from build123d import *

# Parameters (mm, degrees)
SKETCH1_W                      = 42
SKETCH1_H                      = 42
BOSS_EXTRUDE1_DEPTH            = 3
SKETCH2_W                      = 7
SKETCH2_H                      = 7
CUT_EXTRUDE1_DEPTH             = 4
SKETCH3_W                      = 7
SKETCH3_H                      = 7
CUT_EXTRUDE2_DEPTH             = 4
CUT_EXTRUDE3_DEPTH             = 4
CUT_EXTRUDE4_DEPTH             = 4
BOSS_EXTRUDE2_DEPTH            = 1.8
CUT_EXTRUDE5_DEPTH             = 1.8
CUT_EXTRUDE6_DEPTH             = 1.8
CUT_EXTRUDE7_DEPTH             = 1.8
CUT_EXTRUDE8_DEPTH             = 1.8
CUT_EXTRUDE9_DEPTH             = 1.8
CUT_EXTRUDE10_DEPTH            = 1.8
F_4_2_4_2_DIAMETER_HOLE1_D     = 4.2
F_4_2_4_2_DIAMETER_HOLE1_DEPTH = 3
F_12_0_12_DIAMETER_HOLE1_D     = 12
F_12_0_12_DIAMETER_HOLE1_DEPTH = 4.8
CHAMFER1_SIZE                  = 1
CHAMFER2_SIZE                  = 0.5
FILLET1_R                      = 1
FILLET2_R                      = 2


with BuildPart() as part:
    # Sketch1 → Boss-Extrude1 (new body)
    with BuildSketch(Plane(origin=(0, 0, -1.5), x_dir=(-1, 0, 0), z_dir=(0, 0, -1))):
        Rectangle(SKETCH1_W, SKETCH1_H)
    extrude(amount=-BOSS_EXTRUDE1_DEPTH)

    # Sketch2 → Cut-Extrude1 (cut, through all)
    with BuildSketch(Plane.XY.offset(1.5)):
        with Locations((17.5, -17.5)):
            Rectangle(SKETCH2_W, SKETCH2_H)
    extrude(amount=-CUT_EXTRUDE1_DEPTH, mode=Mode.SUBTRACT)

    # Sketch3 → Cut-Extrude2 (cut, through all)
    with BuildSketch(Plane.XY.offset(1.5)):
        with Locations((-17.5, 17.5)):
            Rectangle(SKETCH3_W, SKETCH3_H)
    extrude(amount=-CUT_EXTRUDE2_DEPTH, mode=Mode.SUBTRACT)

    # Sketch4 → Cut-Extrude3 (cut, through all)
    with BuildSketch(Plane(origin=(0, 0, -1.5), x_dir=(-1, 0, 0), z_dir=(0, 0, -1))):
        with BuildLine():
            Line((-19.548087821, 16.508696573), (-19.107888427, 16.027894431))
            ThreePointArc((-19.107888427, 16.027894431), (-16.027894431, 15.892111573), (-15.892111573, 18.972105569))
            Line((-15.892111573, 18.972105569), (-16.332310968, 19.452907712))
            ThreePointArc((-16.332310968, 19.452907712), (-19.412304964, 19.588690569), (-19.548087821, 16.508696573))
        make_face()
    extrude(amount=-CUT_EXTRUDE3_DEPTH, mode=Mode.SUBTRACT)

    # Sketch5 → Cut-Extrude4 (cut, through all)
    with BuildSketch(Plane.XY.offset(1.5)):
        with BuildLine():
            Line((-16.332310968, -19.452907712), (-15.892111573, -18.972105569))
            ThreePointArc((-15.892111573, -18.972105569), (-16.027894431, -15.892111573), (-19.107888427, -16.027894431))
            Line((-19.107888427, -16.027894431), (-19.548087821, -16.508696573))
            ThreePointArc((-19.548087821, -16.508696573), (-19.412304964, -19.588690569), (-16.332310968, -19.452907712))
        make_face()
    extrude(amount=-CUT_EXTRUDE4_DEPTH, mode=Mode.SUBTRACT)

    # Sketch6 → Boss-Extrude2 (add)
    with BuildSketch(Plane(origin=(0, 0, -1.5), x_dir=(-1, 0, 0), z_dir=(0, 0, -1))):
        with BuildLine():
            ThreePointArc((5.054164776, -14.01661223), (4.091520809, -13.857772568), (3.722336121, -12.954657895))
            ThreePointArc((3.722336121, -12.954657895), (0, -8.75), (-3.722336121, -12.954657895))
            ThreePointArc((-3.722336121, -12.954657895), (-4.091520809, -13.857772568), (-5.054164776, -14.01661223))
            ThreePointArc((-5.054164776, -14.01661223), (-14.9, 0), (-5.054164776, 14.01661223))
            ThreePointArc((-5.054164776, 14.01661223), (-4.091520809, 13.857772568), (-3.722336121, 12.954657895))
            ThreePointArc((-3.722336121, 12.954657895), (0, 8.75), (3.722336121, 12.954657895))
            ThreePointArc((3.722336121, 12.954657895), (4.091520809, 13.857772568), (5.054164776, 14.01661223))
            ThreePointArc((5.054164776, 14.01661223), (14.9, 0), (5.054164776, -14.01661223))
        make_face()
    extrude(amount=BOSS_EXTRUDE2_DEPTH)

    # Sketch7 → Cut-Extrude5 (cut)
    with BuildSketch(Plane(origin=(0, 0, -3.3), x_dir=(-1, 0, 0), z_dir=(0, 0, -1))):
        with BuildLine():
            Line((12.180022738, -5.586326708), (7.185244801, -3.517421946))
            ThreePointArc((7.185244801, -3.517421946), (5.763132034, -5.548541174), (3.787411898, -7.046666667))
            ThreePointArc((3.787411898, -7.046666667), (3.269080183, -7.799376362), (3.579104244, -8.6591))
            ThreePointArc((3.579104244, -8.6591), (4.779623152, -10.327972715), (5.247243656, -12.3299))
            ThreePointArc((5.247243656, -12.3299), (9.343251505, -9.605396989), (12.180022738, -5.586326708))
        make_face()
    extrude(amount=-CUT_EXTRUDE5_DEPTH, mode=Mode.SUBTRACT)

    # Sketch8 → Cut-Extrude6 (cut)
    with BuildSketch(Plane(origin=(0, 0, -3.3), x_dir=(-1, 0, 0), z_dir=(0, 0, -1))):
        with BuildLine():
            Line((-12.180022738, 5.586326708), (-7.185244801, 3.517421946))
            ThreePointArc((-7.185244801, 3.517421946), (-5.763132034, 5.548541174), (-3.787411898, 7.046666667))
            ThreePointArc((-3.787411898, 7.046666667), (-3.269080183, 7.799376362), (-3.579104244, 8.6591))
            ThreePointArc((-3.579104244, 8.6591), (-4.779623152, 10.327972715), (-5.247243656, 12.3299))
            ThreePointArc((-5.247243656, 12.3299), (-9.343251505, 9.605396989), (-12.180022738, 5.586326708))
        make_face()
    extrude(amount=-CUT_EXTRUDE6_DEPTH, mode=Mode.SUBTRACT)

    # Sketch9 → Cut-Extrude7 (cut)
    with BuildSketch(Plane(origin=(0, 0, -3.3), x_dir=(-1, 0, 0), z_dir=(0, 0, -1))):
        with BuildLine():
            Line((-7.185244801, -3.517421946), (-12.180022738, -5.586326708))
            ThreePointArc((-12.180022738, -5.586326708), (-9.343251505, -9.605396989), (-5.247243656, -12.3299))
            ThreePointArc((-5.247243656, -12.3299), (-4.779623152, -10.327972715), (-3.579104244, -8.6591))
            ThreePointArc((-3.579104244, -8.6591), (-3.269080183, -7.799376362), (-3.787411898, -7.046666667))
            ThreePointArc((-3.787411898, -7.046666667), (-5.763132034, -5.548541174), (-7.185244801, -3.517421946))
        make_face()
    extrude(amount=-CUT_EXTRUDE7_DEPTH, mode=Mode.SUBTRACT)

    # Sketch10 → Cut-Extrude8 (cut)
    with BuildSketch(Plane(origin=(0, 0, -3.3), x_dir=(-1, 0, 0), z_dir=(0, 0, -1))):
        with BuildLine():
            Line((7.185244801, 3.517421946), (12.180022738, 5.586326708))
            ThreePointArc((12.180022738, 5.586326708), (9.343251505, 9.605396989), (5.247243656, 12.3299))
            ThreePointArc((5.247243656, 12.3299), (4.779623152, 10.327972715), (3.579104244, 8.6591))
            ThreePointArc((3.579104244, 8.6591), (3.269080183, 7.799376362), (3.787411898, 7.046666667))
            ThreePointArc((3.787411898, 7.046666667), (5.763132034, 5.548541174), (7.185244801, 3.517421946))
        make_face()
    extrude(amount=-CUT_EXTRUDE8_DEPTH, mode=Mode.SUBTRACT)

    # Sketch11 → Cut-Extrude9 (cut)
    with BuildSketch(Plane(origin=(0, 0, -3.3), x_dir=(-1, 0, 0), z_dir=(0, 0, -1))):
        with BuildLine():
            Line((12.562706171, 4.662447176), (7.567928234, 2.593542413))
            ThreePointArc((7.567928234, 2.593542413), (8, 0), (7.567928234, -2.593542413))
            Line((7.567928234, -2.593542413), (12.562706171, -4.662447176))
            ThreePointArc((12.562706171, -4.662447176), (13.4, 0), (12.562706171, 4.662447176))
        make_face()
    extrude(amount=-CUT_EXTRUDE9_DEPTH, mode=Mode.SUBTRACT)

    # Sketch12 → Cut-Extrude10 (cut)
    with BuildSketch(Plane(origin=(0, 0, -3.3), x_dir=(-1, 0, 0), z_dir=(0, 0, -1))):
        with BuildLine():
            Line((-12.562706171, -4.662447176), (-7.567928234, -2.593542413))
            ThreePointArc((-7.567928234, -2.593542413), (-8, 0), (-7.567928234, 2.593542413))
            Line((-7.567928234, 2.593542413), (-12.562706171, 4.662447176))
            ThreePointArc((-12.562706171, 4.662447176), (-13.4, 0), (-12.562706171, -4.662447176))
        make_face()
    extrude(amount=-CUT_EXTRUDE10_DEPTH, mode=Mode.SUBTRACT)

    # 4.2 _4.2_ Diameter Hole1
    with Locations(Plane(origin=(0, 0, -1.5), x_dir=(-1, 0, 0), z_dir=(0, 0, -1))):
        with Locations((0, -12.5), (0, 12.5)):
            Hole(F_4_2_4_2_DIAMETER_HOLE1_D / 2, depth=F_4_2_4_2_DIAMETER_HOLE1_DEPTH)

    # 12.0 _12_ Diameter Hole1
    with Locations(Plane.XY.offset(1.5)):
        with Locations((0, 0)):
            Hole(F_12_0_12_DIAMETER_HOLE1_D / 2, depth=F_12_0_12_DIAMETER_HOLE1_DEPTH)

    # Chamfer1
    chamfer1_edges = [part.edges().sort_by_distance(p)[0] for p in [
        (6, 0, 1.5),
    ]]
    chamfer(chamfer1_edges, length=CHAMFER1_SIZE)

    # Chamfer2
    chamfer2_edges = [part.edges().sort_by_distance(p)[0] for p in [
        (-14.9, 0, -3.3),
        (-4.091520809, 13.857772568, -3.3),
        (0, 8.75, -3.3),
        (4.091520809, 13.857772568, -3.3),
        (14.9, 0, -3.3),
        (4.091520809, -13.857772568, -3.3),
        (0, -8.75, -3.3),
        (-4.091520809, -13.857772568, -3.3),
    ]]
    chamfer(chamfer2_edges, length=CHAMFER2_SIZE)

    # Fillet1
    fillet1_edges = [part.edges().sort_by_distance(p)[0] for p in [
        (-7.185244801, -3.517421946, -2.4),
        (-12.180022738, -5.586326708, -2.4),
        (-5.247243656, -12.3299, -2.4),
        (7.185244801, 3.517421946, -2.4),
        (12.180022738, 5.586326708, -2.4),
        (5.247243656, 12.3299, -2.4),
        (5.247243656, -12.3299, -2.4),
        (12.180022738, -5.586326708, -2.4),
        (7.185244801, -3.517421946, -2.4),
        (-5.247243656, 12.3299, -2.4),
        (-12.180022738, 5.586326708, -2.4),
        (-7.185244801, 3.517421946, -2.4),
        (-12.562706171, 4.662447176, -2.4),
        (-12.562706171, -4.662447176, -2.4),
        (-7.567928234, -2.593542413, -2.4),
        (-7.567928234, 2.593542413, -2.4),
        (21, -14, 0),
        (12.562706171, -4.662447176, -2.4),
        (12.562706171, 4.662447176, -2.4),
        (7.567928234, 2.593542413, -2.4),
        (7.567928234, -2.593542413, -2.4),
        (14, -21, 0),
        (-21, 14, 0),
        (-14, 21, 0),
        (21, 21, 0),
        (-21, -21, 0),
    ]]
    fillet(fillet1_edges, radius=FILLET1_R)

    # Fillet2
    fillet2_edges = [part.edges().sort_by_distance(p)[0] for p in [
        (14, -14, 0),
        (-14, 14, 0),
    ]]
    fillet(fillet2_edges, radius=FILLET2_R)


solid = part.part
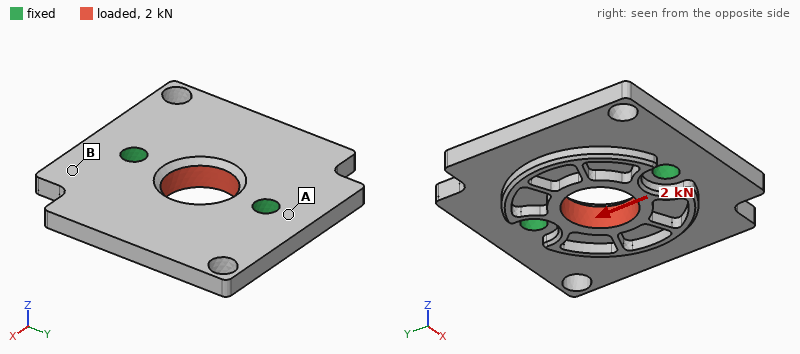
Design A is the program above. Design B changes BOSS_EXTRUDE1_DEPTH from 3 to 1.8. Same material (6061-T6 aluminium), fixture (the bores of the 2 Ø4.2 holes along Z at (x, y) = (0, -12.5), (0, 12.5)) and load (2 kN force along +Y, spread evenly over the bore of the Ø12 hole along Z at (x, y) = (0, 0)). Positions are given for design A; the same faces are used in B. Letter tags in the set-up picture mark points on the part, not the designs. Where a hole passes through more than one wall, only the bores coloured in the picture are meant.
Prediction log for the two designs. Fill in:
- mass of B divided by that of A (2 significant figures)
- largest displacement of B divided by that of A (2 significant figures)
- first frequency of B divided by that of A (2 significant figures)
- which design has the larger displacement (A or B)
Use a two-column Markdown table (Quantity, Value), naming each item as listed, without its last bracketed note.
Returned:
| Quantity | Value |
|---|---|
| mass of B divided by that of A | 0.64 |
| largest displacement of B divided by that of A | 1.7 |
| first frequency of B divided by that of A | 0.69 |
| which design has the larger displacement | B |
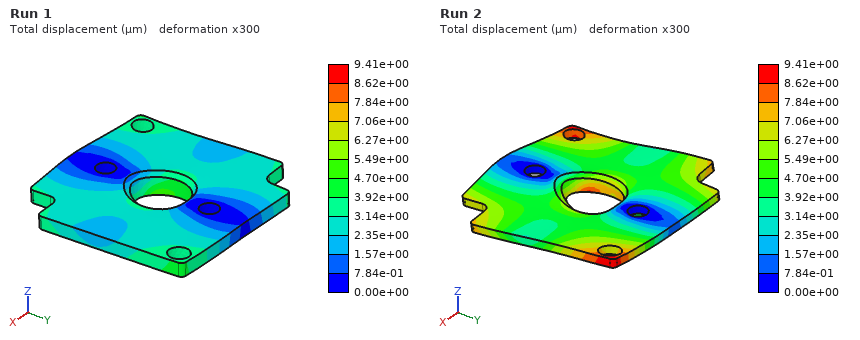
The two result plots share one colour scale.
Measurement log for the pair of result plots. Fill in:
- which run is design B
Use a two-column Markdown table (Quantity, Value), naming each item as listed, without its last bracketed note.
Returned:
| Quantity | Value |
|---|---|
| which run is design B | Run 2 |
